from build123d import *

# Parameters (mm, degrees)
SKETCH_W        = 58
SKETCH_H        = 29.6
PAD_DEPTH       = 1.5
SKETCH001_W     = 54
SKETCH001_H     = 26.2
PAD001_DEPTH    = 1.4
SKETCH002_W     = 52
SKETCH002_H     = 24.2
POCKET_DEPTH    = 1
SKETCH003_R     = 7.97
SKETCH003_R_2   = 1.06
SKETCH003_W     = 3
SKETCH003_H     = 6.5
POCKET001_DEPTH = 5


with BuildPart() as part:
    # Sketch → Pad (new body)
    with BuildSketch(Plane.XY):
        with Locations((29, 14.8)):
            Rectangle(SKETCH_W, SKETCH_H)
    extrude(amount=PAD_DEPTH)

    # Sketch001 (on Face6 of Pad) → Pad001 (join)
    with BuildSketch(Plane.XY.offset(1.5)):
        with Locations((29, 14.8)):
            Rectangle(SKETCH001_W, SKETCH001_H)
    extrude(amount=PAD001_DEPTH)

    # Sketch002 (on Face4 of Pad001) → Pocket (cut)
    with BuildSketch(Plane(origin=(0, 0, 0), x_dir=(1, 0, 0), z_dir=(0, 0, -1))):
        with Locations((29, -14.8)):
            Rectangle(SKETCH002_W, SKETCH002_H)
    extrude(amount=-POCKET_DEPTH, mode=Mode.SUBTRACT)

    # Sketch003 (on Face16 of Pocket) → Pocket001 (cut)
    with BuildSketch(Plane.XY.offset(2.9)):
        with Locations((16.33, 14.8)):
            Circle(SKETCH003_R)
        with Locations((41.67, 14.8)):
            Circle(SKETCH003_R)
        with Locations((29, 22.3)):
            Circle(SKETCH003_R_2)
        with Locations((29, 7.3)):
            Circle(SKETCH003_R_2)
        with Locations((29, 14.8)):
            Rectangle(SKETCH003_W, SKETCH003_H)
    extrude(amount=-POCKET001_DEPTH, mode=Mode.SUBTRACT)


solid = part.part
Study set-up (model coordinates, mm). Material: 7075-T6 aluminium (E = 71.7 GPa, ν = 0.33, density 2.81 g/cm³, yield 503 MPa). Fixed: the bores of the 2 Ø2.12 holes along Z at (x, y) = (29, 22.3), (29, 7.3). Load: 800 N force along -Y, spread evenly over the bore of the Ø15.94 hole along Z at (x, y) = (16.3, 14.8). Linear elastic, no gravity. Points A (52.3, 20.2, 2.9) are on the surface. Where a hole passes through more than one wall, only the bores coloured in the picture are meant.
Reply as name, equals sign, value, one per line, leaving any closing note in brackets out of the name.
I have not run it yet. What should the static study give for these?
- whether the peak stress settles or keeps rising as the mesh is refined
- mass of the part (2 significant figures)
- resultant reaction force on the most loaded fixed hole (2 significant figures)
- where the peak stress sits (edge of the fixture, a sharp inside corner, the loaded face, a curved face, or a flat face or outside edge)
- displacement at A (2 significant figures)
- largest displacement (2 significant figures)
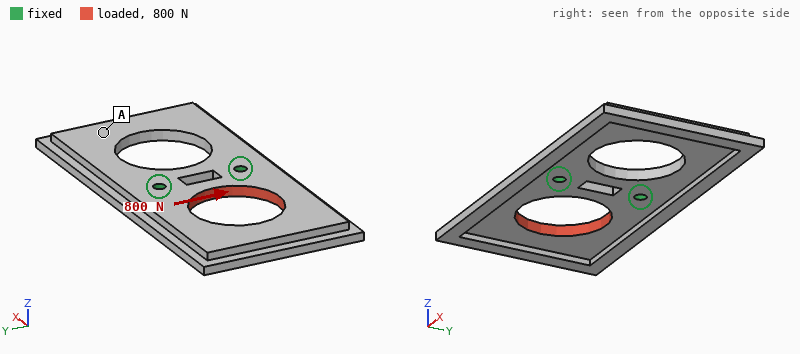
whether the peak stress settles or keeps rising as the mesh is refined = keeps rising
mass of the part = 7.0 g
resultant reaction force on the most loaded fixed hole = 630 N
where the peak stress sits = edge of the fixture
displacement at A = 29 µm
largest displacement = 85 µm
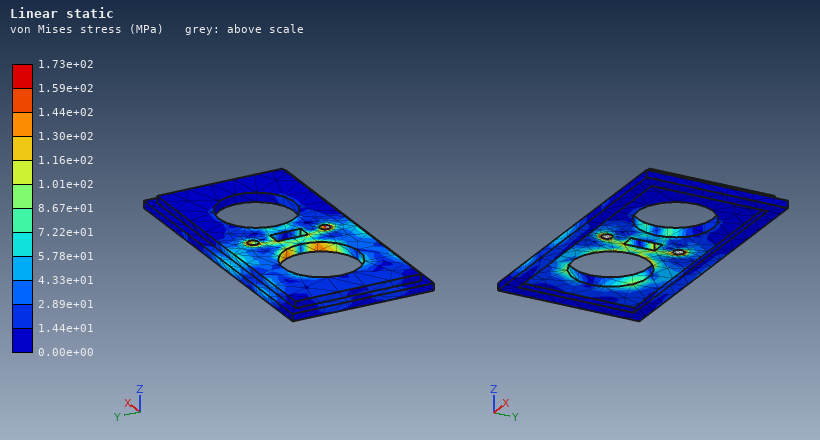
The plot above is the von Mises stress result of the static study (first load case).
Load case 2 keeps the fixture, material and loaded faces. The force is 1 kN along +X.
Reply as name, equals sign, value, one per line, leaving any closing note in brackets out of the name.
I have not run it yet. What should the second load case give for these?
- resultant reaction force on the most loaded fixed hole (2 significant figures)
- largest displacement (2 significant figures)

resultant reaction force on the most loaded fixed hole = 500 N
largest displacement = 29 µm
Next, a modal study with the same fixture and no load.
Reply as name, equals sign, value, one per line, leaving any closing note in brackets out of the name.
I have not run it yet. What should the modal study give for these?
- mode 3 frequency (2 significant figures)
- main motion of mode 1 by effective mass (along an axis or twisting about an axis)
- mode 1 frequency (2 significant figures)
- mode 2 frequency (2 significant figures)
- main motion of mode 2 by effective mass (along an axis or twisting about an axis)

mode 3 frequency = 3500 Hz
main motion of mode 1 by effective mass = twisting about Y
mode 1 frequency = 1700 Hz
mode 2 frequency = 2000 Hz
main motion of mode 2 by effective mass = along Z
